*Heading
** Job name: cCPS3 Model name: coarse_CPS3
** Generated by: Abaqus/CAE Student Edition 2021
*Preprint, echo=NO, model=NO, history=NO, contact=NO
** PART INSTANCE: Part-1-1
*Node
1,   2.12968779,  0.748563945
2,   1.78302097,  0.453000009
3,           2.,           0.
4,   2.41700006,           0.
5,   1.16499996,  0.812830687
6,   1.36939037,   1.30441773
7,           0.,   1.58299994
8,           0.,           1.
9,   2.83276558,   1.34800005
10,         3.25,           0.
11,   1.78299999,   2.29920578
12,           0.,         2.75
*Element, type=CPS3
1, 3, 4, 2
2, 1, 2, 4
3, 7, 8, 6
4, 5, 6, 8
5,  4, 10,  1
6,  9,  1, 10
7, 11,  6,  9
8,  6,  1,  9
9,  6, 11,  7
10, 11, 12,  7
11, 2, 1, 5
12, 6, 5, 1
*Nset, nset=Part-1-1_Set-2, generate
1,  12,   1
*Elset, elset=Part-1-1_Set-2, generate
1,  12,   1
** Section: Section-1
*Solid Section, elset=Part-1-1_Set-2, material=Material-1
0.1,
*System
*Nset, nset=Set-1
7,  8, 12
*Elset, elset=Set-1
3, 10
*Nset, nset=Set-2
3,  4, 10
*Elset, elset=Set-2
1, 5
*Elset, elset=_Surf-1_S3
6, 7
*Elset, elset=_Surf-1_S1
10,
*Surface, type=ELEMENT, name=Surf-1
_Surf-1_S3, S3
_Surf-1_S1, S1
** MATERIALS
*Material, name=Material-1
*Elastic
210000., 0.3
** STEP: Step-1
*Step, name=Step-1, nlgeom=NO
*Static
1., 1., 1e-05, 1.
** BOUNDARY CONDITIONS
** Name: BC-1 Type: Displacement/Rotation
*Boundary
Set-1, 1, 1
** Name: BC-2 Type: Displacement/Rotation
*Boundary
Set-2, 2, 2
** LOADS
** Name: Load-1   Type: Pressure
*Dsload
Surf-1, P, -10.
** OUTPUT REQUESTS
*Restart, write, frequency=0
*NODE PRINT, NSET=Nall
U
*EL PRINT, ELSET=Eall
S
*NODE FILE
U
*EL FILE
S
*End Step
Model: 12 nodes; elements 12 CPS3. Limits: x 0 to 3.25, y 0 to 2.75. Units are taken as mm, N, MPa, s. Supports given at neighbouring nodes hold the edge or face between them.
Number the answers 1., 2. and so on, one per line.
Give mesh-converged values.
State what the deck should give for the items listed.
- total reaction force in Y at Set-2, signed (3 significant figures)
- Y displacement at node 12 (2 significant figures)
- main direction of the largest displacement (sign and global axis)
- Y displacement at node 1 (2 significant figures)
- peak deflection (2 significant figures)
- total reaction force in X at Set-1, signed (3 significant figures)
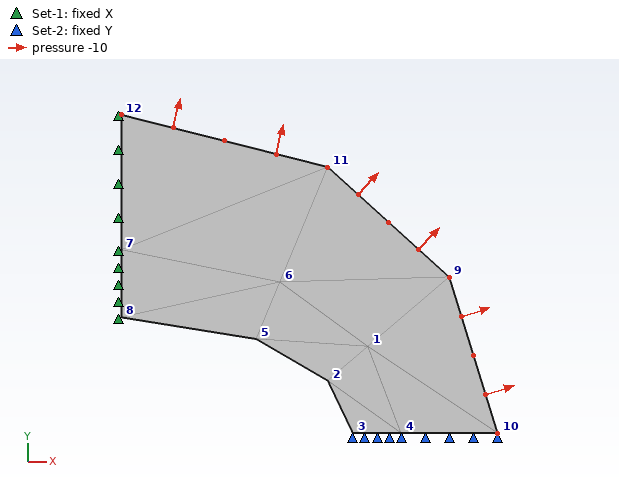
1. -3.25 N
2. 5.5e-04 mm
3. +Y
4. 1.3e-04 mm
5. 5.5e-04 mm
6. -2.75 N
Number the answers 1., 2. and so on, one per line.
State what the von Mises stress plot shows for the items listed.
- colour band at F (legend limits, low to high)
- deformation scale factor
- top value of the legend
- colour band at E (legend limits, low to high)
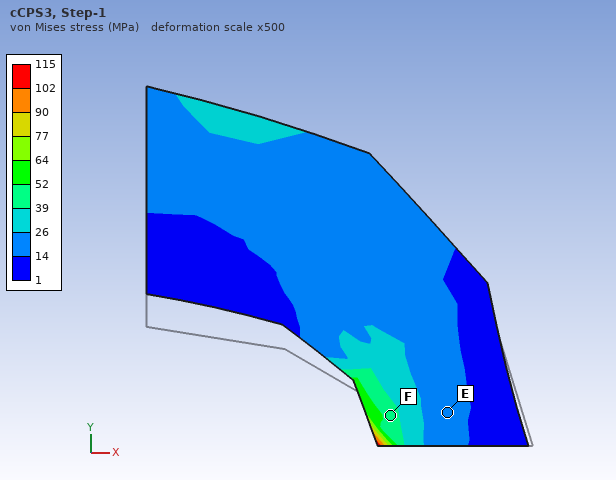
1. 39 to 52 MPa
2. 500
3. 115 MPa
4. 14 to 26 MPa
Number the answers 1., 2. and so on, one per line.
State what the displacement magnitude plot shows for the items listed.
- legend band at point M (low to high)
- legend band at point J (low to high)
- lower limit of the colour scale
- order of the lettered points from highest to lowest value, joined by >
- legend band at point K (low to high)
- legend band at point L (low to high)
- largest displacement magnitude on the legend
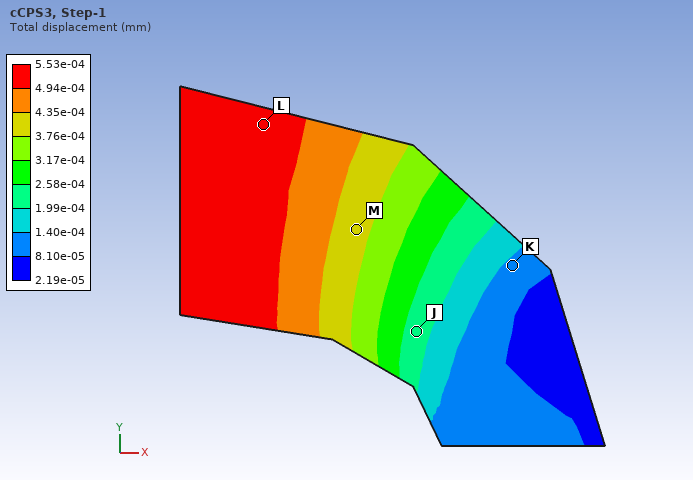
1. 3.76e-04 to 4.35e-04 mm
2. 1.99e-04 to 2.58e-04 mm
3. 2.19e-05 mm
4. L > M > J > K
5. 8.10e-05 to 1.40e-04 mm
6. 4.94e-04 to 5.53e-04 mm
7. 5.53e-04 mm
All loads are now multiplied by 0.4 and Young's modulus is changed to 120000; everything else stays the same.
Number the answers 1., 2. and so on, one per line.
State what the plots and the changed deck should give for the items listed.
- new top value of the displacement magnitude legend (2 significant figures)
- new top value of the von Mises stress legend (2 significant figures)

1. 3.9e-04 mm
2. 46 MPa
